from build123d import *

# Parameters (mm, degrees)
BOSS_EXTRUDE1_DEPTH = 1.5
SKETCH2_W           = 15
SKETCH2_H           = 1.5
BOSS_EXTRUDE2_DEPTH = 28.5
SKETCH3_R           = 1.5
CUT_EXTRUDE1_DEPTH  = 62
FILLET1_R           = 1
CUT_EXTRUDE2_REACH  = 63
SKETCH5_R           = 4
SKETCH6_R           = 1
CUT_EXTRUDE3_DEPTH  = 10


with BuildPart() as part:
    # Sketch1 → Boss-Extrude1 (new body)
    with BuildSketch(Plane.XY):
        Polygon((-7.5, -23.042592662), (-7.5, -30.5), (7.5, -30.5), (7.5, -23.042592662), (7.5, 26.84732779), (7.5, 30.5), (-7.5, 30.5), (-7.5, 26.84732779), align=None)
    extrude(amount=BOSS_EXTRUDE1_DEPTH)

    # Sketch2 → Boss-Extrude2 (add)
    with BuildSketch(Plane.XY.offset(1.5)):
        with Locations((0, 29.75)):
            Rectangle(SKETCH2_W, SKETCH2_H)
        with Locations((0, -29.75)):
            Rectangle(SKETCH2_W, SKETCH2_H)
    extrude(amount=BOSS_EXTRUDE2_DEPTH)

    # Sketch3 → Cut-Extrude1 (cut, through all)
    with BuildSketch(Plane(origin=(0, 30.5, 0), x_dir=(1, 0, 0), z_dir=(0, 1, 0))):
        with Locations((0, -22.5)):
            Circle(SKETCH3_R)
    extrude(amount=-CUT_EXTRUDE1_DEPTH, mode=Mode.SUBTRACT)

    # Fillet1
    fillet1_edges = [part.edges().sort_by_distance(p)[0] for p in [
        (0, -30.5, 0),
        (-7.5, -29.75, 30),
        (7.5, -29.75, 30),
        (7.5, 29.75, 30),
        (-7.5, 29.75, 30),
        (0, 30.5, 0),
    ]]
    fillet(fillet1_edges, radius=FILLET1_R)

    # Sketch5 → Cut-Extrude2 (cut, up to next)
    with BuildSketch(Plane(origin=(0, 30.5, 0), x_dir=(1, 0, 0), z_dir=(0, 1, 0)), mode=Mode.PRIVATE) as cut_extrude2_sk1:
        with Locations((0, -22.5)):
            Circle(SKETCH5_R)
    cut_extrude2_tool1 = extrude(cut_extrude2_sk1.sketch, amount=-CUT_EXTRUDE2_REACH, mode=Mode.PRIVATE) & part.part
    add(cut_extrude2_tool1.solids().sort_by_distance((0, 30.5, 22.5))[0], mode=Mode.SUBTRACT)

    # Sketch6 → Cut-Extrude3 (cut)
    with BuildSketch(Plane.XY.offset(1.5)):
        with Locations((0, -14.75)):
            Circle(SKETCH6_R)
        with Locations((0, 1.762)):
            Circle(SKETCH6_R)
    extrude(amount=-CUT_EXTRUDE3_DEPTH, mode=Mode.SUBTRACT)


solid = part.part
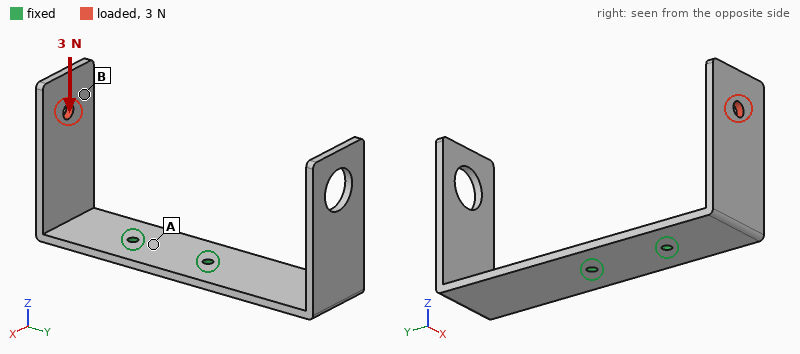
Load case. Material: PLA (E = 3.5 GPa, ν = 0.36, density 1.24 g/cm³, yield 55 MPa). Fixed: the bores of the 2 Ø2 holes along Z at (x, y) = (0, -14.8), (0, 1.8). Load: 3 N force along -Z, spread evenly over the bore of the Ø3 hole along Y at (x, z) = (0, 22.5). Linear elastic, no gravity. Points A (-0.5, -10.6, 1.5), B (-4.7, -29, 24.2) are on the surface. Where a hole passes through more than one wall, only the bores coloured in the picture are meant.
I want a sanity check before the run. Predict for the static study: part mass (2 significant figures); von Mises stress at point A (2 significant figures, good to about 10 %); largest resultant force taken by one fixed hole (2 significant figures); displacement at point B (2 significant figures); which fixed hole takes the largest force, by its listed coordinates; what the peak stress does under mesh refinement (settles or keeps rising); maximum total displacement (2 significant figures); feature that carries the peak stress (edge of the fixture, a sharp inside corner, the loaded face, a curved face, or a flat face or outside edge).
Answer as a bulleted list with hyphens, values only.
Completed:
- 3.2 g
- 1.3 MPa
- 3.7 N
- 0.57 mm
- (0, -14.8)
- keeps rising
- 0.71 mm
- edge of the fixture
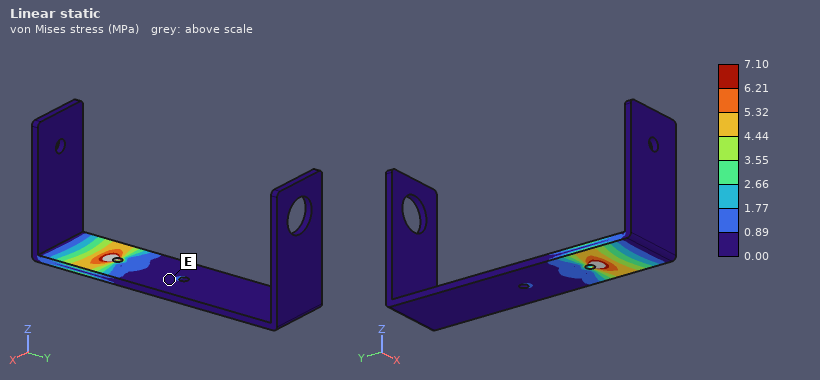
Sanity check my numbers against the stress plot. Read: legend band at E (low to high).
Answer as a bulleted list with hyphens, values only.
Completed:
- 0.00 to 0.89 MPa
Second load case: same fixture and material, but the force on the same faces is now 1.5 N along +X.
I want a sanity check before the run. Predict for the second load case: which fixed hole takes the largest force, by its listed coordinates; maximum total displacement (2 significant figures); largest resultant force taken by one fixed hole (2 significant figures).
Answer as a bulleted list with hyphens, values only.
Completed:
- (0, -14.8)
- 0.63 mm
- 2.7 N
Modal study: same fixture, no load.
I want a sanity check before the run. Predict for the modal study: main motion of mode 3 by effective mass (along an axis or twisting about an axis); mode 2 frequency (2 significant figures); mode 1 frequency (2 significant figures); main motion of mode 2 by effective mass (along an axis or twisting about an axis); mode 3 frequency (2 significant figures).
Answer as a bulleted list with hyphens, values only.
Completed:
- along X
- 270 Hz
- 180 Hz
- along Y
- 310 Hz
